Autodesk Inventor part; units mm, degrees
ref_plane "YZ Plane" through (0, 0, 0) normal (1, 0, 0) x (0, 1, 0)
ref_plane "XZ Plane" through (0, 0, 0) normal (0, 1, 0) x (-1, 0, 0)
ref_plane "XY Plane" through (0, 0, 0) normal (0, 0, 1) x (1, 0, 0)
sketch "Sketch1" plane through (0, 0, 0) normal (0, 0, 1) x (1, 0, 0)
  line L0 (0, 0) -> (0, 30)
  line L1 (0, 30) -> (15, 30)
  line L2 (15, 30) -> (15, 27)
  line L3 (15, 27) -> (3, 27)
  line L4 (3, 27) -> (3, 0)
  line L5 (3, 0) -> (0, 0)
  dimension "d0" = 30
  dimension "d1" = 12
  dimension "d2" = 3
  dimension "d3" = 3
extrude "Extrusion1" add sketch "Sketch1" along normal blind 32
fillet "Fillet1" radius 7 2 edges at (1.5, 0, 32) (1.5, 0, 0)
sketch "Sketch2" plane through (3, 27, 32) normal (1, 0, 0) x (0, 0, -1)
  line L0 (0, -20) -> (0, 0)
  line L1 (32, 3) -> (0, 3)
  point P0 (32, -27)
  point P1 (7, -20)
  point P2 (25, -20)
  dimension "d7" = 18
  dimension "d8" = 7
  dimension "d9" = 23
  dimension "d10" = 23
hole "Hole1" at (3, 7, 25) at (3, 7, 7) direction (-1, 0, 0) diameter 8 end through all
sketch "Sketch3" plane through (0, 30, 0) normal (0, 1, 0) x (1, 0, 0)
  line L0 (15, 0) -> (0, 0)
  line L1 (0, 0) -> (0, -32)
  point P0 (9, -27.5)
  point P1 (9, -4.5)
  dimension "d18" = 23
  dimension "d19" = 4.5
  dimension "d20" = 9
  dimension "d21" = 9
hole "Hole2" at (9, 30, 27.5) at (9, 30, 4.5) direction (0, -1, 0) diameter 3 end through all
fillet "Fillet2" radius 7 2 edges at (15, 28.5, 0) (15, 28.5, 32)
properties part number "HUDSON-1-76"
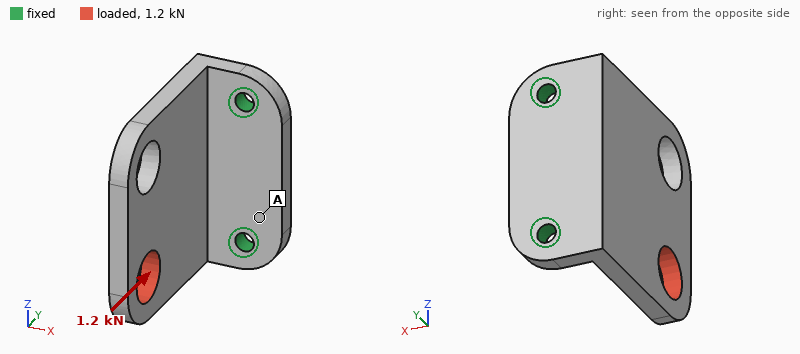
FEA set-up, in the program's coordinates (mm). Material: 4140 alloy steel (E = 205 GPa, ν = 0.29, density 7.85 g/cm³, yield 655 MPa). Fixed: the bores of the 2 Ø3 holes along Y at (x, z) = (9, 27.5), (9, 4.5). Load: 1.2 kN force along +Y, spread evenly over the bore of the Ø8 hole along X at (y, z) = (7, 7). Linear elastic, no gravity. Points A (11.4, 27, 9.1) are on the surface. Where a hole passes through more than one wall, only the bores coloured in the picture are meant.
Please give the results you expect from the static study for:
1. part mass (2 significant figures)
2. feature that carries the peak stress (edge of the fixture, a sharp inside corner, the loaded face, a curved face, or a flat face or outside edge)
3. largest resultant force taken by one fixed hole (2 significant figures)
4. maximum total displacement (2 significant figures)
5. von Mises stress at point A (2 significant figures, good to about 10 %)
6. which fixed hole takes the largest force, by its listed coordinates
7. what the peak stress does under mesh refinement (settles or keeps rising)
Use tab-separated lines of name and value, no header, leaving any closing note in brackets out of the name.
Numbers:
part mass	28 g
feature that carries the peak stress	edge of the fixture
largest resultant force taken by one fixed hole	1.1 kN
maximum total displacement	88 µm
von Mises stress at point A	48 MPa
which fixed hole takes the largest force, by its listed coordinates	(9, 4.5)
what the peak stress does under mesh refinement	keeps rising
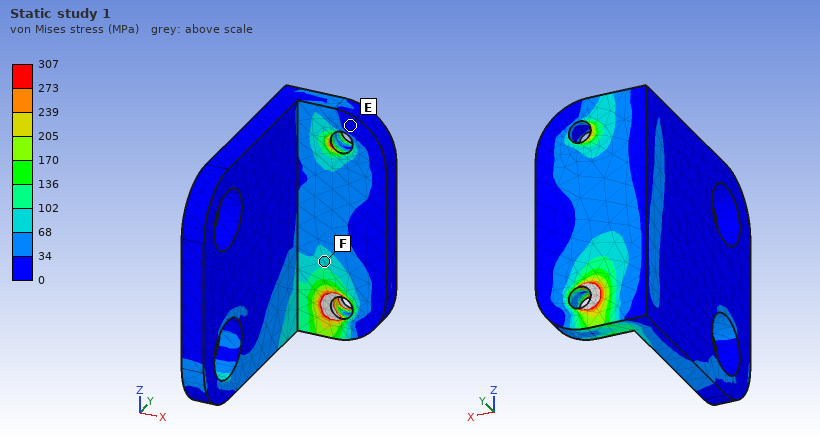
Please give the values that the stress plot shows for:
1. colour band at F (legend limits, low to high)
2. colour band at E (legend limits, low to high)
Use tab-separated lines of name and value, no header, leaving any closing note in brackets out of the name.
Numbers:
colour band at F	68 to 102 MPa
colour band at E	0 to 34 MPa
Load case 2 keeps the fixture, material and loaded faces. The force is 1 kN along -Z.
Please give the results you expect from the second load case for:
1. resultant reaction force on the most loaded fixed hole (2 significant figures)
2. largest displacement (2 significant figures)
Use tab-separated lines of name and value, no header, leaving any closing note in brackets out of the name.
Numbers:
resultant reaction force on the most loaded fixed hole	1.1 kN
largest displacement	51 µm
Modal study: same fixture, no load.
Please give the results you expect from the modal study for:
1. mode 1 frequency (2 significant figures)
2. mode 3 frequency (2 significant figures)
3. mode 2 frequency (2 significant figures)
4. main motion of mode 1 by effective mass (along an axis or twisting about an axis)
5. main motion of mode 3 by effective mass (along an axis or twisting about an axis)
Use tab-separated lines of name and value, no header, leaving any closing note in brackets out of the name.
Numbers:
mode 1 frequency	2500 Hz
mode 3 frequency	9300 Hz
mode 2 frequency	6400 Hz
main motion of mode 1 by effective mass	along X
main motion of mode 3 by effective mass	along Z
